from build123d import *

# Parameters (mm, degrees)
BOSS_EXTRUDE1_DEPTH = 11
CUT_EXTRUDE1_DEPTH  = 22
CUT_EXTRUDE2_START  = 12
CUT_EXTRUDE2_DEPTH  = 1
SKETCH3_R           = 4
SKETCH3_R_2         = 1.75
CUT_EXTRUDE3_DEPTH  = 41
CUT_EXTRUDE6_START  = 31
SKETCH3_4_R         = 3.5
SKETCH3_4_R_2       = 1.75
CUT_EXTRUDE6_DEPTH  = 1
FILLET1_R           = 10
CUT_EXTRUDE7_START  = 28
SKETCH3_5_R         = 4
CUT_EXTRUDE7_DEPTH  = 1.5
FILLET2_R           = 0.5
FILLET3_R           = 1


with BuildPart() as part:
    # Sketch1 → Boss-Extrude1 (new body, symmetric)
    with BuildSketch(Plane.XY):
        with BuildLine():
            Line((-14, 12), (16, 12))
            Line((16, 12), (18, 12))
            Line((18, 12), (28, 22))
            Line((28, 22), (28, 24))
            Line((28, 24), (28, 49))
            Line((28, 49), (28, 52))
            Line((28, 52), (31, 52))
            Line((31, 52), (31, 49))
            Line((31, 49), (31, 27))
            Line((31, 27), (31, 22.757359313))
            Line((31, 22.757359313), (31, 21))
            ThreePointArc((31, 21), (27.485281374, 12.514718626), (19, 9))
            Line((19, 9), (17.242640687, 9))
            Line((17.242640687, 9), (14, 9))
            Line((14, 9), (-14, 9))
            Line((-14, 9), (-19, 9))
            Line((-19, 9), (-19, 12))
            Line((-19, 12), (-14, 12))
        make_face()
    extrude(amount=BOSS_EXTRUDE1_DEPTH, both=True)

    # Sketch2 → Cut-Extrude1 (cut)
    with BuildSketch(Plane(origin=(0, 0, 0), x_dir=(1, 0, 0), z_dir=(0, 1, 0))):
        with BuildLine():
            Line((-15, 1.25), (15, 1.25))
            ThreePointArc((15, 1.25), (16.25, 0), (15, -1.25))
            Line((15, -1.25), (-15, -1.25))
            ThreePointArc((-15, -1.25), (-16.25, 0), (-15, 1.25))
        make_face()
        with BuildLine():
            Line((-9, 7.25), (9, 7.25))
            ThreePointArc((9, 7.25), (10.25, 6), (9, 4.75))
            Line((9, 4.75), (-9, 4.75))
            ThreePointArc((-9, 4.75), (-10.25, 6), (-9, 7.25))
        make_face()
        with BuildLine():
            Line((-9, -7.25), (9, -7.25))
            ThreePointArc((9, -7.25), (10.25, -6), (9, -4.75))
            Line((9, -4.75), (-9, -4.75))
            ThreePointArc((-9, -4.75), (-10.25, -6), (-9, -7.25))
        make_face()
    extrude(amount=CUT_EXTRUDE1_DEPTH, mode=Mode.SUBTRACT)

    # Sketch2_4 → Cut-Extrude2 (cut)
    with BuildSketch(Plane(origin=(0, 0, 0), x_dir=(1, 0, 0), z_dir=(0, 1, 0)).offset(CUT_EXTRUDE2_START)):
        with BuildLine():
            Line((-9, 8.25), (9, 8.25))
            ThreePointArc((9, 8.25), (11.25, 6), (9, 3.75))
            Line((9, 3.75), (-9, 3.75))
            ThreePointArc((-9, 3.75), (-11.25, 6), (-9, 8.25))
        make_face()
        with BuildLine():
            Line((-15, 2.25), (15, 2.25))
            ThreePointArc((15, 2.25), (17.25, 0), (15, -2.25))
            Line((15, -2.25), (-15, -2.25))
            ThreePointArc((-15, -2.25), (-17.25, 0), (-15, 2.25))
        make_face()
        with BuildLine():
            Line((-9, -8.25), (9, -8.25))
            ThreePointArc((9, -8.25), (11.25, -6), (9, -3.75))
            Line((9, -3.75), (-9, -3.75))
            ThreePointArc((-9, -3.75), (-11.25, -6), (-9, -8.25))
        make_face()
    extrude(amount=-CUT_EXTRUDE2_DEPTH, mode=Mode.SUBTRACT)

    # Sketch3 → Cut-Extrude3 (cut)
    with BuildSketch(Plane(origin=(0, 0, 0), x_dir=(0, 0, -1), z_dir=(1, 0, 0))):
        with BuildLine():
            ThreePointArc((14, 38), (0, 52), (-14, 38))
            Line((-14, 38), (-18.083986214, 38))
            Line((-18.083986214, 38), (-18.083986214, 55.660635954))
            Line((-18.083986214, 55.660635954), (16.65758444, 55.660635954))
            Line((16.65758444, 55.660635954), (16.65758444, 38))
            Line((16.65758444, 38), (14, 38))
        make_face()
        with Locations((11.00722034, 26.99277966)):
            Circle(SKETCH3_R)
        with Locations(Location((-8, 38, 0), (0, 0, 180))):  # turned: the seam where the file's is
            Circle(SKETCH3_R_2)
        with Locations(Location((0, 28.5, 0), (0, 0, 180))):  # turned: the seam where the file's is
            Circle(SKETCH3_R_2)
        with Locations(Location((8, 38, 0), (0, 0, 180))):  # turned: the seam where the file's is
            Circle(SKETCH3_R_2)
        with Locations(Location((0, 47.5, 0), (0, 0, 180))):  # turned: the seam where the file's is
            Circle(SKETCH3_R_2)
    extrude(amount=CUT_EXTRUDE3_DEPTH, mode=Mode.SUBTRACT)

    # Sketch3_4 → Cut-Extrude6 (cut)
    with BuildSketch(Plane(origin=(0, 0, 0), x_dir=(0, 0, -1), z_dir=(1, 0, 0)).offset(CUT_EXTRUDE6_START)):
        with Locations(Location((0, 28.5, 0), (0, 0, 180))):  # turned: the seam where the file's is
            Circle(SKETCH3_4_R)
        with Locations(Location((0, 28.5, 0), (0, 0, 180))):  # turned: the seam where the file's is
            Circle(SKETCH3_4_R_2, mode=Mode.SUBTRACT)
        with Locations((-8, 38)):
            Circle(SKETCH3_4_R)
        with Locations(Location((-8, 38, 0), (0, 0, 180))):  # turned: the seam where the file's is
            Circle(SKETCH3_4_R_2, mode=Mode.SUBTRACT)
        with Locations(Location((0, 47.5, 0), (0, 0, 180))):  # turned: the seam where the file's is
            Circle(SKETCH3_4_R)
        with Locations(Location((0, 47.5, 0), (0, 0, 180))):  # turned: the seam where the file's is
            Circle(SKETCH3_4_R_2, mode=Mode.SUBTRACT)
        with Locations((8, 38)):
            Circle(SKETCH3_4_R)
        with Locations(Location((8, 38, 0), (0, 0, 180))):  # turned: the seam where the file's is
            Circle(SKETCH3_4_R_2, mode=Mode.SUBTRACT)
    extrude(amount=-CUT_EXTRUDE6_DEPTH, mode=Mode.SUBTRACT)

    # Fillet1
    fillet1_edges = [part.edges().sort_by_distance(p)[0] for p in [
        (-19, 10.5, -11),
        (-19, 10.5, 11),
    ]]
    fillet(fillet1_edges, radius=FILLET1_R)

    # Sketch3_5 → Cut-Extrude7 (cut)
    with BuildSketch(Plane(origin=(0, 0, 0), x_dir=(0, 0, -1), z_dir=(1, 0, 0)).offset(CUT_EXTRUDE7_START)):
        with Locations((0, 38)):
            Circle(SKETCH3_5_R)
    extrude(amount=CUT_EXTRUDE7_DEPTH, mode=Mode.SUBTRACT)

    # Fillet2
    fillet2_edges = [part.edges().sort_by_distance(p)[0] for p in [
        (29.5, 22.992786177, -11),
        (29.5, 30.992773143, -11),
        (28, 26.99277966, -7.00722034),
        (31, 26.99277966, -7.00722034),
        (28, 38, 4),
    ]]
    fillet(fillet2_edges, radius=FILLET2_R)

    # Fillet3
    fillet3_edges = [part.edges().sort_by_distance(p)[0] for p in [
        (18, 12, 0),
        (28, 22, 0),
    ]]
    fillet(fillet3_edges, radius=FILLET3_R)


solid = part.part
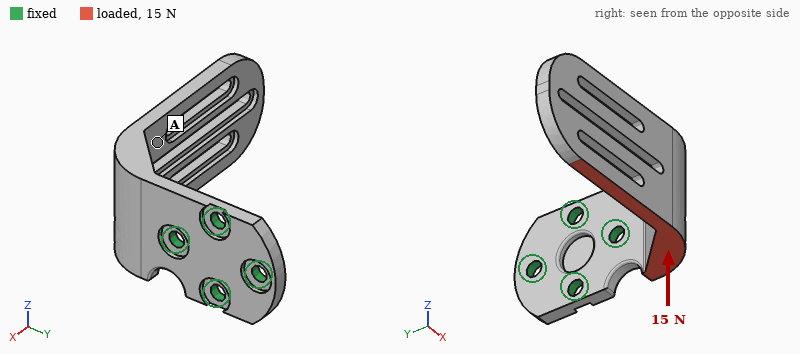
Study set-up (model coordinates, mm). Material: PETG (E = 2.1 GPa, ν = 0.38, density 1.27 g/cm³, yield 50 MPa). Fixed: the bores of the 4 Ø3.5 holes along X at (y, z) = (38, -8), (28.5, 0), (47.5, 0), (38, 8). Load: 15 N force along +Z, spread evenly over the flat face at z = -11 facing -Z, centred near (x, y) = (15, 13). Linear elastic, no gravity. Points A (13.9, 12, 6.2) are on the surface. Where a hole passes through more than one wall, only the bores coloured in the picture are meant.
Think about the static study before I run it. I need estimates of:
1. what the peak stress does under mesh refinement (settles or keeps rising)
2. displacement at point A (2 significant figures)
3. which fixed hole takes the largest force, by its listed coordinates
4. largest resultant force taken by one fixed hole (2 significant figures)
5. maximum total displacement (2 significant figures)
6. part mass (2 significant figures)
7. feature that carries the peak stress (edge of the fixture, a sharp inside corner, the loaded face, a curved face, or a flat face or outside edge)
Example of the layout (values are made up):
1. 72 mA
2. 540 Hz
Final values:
1. keeps rising
2. 0.25 mm
3. (28.5, 0)
4. 27 N
5. 0.75 mm
6. 6.4 g
7. edge of the fixture
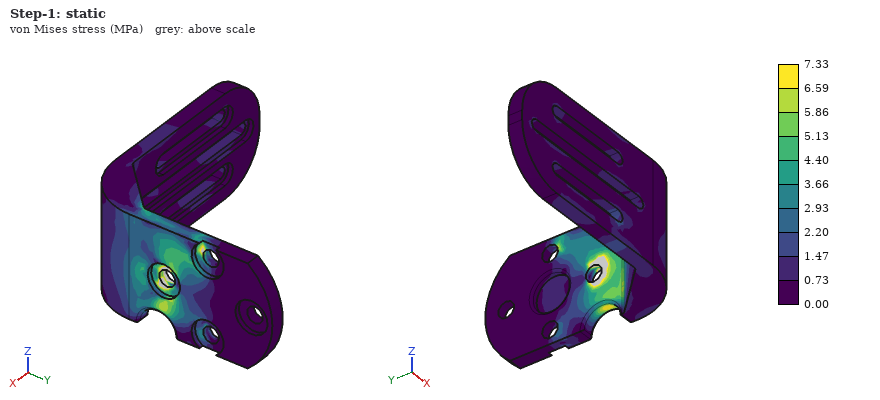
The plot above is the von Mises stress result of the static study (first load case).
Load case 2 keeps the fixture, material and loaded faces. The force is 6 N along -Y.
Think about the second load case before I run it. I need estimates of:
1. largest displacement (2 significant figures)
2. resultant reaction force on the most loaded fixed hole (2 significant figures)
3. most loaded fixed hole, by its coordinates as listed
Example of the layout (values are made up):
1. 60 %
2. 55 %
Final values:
1. 0.68 mm
2. 13 N
3. (28.5, 0)
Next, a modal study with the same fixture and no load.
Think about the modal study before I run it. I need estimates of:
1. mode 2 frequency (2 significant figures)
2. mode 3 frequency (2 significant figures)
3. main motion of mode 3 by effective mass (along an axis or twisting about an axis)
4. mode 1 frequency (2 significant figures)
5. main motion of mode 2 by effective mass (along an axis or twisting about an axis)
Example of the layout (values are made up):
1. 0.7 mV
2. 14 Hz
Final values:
1. 390 Hz
2. 790 Hz
3. along X
4. 250 Hz
5. along Z
